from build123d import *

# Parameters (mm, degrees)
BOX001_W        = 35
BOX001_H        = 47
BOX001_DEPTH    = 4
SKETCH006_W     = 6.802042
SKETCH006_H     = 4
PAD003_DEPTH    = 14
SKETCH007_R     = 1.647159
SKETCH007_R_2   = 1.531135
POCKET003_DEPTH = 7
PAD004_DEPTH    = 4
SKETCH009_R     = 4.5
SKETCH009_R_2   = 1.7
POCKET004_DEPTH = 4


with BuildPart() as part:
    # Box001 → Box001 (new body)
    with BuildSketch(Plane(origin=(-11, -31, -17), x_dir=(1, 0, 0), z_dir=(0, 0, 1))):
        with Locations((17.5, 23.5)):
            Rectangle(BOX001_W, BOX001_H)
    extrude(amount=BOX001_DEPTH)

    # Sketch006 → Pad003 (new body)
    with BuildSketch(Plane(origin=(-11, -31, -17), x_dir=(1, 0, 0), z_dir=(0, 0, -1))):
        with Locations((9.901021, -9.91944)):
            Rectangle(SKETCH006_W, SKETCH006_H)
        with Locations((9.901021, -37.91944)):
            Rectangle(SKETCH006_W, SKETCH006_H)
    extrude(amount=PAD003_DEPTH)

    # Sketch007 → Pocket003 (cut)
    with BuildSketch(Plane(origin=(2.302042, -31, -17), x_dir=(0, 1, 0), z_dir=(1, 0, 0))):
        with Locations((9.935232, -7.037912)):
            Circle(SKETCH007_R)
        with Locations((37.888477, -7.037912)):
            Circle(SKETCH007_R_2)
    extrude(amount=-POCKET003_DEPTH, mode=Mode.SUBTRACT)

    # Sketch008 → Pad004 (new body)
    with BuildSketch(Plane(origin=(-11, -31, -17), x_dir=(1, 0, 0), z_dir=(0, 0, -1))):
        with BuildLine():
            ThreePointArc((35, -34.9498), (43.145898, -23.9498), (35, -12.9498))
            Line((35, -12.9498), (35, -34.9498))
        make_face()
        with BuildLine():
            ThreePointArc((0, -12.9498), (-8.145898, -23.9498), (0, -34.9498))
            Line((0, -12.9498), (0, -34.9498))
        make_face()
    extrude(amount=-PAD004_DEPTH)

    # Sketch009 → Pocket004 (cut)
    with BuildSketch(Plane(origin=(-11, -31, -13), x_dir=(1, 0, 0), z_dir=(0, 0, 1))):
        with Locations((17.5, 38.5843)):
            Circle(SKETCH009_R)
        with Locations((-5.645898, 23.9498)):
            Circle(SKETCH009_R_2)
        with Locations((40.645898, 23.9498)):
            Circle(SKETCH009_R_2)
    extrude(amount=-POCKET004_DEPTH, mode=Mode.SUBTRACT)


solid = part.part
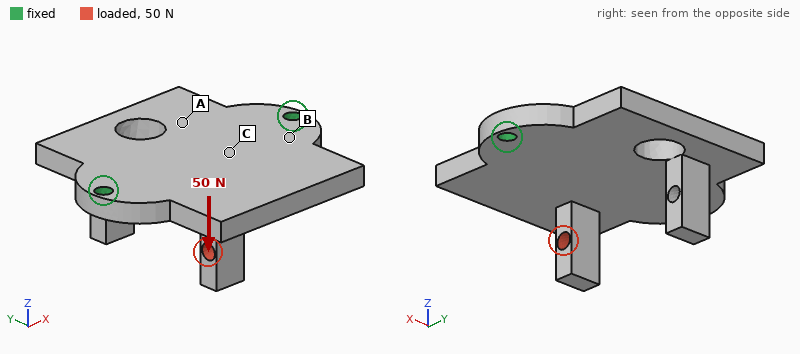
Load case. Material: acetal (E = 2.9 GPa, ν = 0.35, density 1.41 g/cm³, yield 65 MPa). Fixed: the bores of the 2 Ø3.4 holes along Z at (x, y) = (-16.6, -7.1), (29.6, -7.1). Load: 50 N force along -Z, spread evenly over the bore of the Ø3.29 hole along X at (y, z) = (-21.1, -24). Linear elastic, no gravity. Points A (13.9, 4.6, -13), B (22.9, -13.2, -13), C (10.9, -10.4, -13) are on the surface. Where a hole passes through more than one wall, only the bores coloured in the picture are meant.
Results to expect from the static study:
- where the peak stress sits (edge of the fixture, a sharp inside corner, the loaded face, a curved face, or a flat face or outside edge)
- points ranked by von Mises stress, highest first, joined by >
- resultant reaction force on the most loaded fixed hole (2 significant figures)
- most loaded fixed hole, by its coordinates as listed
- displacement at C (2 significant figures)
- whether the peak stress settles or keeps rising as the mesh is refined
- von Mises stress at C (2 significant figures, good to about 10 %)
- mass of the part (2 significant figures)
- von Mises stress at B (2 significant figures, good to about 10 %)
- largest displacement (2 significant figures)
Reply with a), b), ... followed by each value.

a) edge of the fixture
b) B > C > A
c) 35 N
d) (-16.6, -7.1)
e) 0.085 mm
f) keeps rising
g) 3.0 MPa
h) 11 g
i) 4.6 MPa
j) 0.41 mm
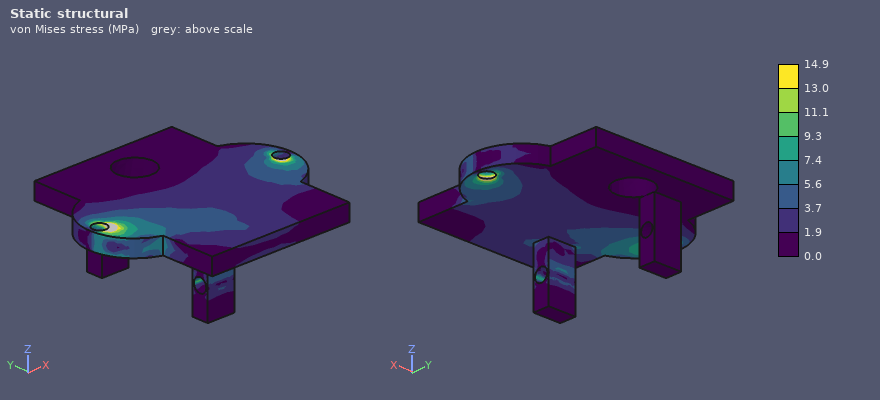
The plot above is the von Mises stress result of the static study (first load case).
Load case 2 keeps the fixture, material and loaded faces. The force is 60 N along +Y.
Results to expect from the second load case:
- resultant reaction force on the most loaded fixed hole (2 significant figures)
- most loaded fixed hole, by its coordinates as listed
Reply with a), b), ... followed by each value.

a) 41 N
b) (-16.6, -7.1)
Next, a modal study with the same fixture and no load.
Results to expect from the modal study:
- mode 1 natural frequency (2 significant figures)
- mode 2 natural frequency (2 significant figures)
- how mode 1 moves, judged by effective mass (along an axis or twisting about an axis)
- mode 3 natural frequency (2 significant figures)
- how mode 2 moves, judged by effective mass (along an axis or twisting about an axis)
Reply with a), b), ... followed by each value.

a) 930 Hz
b) 1300 Hz
c) twisting about X
d) 2500 Hz
e) along Z
